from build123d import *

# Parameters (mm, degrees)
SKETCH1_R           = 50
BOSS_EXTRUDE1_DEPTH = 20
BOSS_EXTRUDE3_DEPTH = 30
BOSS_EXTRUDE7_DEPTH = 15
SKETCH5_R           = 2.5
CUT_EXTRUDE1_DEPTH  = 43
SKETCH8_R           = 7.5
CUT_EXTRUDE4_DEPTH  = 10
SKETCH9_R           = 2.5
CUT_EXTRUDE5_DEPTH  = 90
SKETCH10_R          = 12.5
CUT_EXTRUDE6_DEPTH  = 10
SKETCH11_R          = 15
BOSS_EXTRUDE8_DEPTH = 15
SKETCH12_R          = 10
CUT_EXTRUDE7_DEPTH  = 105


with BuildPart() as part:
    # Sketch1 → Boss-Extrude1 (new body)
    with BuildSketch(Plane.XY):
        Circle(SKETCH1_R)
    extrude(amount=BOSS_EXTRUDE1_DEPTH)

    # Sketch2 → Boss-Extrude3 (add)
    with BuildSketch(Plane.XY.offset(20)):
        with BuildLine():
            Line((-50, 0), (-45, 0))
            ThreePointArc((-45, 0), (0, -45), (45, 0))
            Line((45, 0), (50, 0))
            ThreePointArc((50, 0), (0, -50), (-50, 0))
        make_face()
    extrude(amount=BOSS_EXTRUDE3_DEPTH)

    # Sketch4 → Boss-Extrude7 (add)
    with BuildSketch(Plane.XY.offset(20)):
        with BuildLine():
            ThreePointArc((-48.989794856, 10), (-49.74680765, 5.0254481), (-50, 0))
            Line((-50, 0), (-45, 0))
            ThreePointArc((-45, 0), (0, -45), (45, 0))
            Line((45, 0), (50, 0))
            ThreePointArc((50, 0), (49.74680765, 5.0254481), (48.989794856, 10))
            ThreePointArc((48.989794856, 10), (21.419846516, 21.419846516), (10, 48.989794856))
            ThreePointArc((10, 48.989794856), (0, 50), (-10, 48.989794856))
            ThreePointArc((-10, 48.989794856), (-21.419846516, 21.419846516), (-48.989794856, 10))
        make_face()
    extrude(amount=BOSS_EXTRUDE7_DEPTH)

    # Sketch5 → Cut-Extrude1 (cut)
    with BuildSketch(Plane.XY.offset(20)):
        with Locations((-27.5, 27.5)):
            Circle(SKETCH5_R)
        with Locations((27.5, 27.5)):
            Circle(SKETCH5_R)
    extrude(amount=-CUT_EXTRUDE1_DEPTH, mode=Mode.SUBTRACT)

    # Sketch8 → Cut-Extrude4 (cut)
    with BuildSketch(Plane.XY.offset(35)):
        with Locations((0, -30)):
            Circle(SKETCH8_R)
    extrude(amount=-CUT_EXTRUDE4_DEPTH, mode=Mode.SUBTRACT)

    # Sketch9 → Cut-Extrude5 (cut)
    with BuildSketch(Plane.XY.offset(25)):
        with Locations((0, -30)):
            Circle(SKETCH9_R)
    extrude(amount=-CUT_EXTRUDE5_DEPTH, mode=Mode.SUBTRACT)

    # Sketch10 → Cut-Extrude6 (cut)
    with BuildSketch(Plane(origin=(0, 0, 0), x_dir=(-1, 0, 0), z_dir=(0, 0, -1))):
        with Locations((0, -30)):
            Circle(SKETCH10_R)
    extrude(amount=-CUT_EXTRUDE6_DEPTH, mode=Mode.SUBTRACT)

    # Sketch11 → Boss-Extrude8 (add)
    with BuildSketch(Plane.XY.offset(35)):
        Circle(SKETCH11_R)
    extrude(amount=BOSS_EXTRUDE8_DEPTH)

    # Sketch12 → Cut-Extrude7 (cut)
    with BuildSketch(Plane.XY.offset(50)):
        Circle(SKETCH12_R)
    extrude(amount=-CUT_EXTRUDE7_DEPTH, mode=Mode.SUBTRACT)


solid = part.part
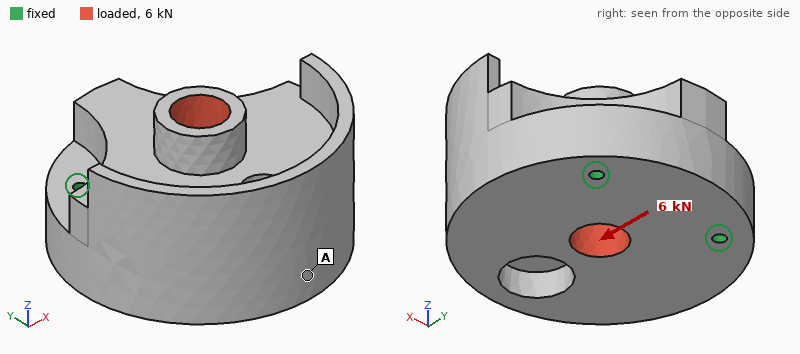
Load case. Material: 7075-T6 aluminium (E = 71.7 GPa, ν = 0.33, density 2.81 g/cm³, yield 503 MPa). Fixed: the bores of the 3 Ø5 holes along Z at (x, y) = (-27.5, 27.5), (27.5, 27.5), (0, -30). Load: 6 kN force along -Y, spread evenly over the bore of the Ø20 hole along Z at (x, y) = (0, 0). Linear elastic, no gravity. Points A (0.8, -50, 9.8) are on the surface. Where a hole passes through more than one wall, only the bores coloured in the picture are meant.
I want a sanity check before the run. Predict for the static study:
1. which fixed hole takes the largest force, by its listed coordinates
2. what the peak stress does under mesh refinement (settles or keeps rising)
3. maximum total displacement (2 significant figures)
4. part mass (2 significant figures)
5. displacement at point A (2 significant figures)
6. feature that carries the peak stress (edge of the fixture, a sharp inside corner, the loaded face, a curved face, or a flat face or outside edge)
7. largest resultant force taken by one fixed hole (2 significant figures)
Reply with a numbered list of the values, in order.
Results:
1. (0, -30)
2. keeps rising
3. 7.5 µm
4. 710 g
5. 1.2 µm
6. edge of the fixture
7. 2.7 kN
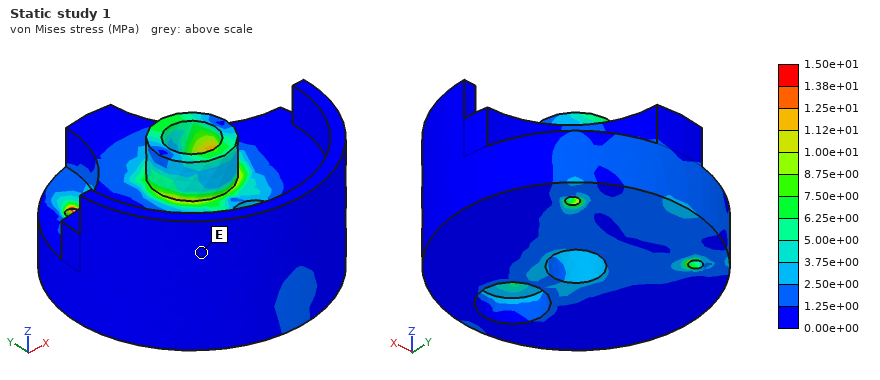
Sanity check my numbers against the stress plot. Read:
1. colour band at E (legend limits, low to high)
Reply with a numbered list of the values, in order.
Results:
1. 0.00e+00 to 1.25e+00 MPa
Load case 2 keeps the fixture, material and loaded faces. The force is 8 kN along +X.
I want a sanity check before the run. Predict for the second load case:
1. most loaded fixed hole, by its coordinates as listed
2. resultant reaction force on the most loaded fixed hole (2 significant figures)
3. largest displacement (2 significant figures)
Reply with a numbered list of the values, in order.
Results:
1. (0, -30)
2. 3.4 kN
3. 12 µm
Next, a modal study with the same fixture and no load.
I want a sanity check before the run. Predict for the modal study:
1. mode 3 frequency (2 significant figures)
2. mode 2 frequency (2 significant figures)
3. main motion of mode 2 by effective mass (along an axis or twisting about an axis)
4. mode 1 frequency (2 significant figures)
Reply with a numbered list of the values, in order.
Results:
1. 11 kHz
2. 8000 Hz
3. along Z
4. 6000 Hz
